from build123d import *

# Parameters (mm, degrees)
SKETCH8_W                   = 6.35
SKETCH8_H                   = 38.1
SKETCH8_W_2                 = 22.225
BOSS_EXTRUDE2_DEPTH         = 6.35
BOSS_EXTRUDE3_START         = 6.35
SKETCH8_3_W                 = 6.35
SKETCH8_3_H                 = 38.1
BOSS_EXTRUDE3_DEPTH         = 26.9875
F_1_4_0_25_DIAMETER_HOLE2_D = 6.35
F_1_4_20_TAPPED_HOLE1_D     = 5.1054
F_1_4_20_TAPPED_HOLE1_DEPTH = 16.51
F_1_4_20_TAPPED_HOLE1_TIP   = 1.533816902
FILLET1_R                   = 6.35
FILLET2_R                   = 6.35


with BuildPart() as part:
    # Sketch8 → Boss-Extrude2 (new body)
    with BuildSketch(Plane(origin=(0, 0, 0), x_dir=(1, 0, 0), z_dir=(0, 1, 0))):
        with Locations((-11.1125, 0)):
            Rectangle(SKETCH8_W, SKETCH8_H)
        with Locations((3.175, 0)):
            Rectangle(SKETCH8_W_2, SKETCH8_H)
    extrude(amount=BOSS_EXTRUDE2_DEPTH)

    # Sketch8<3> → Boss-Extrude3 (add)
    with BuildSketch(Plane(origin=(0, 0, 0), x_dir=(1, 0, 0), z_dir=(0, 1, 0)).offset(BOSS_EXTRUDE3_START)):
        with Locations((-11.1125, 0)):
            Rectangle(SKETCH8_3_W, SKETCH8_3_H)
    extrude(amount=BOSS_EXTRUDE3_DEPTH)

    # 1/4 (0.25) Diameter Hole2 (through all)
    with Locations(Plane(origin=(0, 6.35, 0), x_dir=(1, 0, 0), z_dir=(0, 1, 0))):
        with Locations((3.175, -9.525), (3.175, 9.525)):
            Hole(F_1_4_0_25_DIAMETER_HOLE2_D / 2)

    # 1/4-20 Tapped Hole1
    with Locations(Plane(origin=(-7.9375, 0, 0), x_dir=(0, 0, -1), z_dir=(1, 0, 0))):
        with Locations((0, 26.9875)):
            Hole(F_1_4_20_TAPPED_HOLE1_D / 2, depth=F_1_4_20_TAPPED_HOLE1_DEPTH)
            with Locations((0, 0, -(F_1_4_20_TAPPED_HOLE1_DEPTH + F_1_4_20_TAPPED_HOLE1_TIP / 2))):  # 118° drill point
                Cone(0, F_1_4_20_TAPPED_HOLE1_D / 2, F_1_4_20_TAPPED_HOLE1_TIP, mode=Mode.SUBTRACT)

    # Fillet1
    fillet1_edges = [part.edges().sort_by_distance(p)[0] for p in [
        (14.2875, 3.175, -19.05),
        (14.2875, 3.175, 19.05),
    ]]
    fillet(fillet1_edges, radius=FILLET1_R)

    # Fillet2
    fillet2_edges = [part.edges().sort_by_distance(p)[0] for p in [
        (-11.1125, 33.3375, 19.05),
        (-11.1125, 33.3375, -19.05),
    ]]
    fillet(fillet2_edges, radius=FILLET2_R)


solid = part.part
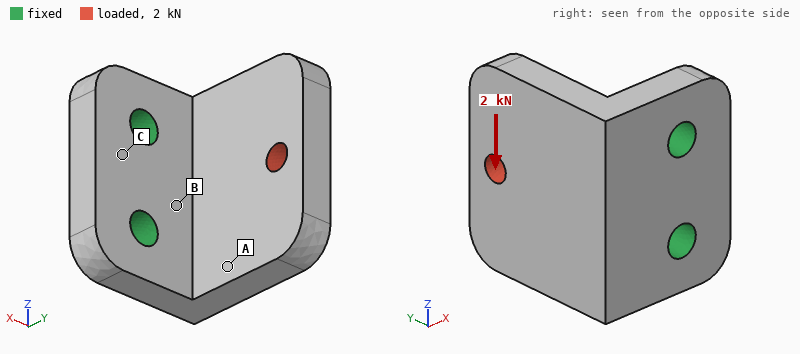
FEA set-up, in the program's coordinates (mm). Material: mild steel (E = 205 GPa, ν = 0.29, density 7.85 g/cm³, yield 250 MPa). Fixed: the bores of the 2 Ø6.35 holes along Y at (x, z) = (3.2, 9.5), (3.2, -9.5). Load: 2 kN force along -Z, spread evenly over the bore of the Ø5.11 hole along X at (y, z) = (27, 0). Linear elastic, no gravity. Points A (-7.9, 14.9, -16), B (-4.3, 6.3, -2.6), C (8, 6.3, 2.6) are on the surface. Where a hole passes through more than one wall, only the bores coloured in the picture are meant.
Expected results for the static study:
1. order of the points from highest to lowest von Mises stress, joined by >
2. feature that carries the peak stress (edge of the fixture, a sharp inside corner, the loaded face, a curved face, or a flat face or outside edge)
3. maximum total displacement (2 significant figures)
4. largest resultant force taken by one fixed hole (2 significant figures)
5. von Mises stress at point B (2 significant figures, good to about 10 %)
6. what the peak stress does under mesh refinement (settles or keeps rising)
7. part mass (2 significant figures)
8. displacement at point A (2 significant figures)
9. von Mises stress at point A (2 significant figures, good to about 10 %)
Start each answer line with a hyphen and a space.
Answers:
- B > A > C
- edge of the fixture
- 36 µm
- 2.4 kN
- 79 MPa
- keeps rising
- 100 g
- 20 µm
- 38 MPa
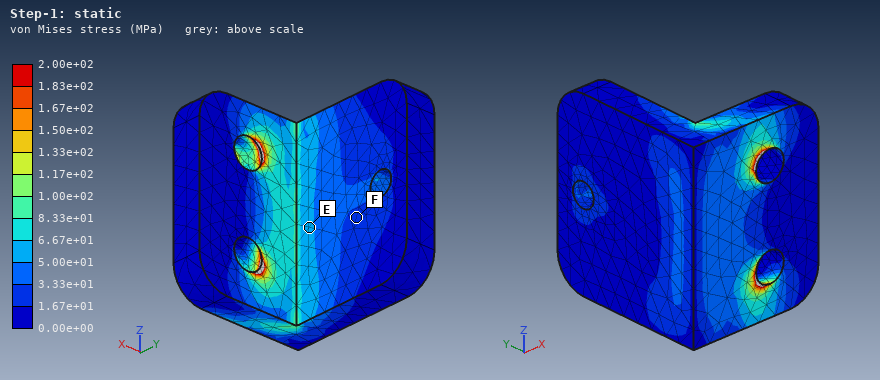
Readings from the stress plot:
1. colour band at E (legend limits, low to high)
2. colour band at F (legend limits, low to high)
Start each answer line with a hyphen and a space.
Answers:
- 5.00e+01 to 6.67e+01 MPa
- 1.67e+01 to 3.33e+01 MPa
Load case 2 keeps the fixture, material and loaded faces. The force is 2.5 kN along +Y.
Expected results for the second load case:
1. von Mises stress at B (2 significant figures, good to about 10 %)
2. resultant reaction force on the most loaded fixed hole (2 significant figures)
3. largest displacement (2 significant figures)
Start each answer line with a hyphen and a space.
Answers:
- 55 MPa
- 1.3 kN
- 44 µm
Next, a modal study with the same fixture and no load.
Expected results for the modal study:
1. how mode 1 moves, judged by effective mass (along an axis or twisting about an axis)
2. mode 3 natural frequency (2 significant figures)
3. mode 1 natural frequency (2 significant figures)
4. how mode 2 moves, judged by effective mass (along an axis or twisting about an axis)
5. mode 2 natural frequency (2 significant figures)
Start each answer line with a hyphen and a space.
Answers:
- along X
- 11 kHz
- 3700 Hz
- along Z
- 6900 Hz
